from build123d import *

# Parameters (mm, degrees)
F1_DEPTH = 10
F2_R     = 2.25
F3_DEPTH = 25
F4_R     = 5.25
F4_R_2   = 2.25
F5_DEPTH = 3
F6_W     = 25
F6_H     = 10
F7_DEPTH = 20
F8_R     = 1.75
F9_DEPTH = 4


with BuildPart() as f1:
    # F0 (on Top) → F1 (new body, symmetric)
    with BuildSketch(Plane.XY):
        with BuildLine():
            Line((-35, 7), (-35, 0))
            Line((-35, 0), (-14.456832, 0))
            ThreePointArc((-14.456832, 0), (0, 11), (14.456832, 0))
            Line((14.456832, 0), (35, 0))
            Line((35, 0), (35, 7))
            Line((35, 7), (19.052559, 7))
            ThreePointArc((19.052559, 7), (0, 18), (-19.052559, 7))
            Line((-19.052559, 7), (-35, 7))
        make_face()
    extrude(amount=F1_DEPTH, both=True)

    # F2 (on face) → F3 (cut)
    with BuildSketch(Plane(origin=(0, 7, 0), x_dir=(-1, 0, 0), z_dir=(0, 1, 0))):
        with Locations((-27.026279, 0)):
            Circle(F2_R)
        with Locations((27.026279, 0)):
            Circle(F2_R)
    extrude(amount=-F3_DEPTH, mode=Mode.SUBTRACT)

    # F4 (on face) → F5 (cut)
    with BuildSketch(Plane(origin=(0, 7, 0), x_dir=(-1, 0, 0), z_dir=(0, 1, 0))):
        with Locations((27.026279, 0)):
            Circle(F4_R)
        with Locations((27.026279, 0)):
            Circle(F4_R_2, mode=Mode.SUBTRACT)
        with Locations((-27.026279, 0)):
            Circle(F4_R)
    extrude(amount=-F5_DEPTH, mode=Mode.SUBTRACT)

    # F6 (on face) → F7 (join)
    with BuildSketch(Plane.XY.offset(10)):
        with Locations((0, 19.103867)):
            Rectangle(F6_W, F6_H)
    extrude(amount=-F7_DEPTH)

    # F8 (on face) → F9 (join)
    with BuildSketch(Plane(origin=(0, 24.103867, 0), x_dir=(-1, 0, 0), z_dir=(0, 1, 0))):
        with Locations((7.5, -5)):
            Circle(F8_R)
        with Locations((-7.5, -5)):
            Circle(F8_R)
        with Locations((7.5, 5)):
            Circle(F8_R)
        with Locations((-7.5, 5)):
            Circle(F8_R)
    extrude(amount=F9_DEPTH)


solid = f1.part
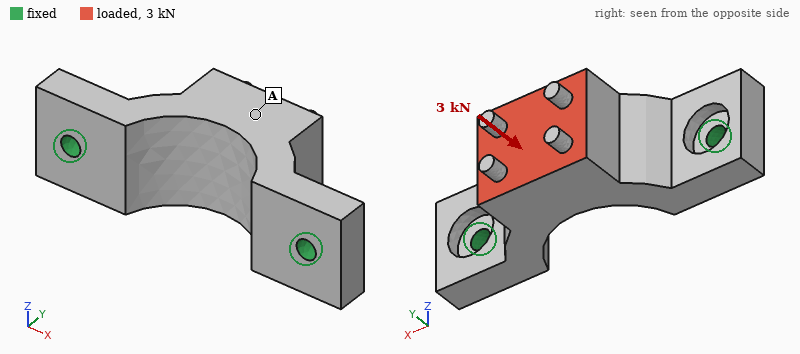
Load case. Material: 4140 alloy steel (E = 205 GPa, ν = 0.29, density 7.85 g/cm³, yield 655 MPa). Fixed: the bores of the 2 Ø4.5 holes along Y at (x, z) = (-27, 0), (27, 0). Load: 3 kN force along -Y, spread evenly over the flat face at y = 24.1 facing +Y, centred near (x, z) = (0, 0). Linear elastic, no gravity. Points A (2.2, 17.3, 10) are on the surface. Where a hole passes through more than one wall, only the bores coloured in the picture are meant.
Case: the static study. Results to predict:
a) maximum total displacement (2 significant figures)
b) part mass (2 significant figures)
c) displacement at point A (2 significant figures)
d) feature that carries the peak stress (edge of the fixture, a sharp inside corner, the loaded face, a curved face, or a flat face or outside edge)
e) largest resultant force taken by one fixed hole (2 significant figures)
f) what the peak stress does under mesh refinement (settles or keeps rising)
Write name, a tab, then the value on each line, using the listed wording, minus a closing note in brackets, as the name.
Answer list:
maximum total displacement	7.7 µm
part mass	110 g
displacement at point A	7.5 µm
feature that carries the peak stress	edge of the fixture
largest resultant force taken by one fixed hole	2.3 kN
what the peak stress does under mesh refinement	keeps rising
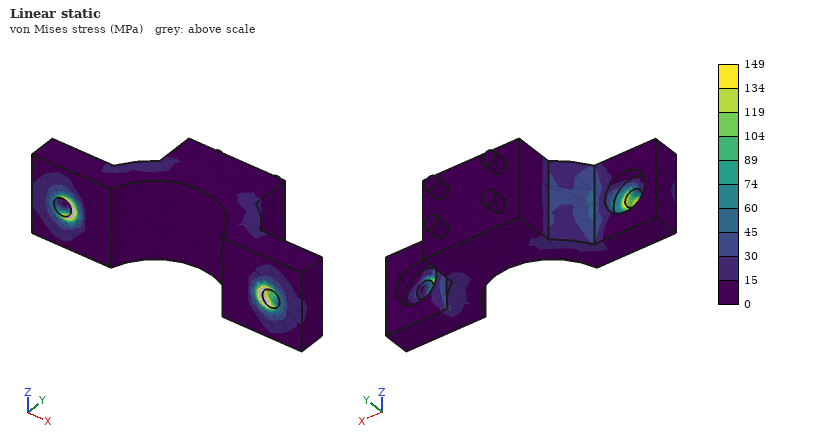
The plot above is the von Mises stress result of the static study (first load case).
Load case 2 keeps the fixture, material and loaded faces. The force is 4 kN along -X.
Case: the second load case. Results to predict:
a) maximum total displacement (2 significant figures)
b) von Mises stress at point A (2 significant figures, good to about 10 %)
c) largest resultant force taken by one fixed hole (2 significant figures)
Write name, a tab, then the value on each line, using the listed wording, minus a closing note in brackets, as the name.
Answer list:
maximum total displacement	13 µm
von Mises stress at point A	16 MPa
largest resultant force taken by one fixed hole	2.7 kN
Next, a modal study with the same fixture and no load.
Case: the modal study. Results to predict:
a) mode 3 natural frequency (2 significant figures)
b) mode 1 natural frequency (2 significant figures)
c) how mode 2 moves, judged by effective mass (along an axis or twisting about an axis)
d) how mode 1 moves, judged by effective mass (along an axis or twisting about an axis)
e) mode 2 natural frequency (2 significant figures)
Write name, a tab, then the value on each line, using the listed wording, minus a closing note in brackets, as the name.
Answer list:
mode 3 natural frequency	15 kHz
mode 1 natural frequency	4100 Hz
how mode 2 moves, judged by effective mass	along Y
how mode 1 moves, judged by effective mass	along Z
mode 2 natural frequency	11 kHz
